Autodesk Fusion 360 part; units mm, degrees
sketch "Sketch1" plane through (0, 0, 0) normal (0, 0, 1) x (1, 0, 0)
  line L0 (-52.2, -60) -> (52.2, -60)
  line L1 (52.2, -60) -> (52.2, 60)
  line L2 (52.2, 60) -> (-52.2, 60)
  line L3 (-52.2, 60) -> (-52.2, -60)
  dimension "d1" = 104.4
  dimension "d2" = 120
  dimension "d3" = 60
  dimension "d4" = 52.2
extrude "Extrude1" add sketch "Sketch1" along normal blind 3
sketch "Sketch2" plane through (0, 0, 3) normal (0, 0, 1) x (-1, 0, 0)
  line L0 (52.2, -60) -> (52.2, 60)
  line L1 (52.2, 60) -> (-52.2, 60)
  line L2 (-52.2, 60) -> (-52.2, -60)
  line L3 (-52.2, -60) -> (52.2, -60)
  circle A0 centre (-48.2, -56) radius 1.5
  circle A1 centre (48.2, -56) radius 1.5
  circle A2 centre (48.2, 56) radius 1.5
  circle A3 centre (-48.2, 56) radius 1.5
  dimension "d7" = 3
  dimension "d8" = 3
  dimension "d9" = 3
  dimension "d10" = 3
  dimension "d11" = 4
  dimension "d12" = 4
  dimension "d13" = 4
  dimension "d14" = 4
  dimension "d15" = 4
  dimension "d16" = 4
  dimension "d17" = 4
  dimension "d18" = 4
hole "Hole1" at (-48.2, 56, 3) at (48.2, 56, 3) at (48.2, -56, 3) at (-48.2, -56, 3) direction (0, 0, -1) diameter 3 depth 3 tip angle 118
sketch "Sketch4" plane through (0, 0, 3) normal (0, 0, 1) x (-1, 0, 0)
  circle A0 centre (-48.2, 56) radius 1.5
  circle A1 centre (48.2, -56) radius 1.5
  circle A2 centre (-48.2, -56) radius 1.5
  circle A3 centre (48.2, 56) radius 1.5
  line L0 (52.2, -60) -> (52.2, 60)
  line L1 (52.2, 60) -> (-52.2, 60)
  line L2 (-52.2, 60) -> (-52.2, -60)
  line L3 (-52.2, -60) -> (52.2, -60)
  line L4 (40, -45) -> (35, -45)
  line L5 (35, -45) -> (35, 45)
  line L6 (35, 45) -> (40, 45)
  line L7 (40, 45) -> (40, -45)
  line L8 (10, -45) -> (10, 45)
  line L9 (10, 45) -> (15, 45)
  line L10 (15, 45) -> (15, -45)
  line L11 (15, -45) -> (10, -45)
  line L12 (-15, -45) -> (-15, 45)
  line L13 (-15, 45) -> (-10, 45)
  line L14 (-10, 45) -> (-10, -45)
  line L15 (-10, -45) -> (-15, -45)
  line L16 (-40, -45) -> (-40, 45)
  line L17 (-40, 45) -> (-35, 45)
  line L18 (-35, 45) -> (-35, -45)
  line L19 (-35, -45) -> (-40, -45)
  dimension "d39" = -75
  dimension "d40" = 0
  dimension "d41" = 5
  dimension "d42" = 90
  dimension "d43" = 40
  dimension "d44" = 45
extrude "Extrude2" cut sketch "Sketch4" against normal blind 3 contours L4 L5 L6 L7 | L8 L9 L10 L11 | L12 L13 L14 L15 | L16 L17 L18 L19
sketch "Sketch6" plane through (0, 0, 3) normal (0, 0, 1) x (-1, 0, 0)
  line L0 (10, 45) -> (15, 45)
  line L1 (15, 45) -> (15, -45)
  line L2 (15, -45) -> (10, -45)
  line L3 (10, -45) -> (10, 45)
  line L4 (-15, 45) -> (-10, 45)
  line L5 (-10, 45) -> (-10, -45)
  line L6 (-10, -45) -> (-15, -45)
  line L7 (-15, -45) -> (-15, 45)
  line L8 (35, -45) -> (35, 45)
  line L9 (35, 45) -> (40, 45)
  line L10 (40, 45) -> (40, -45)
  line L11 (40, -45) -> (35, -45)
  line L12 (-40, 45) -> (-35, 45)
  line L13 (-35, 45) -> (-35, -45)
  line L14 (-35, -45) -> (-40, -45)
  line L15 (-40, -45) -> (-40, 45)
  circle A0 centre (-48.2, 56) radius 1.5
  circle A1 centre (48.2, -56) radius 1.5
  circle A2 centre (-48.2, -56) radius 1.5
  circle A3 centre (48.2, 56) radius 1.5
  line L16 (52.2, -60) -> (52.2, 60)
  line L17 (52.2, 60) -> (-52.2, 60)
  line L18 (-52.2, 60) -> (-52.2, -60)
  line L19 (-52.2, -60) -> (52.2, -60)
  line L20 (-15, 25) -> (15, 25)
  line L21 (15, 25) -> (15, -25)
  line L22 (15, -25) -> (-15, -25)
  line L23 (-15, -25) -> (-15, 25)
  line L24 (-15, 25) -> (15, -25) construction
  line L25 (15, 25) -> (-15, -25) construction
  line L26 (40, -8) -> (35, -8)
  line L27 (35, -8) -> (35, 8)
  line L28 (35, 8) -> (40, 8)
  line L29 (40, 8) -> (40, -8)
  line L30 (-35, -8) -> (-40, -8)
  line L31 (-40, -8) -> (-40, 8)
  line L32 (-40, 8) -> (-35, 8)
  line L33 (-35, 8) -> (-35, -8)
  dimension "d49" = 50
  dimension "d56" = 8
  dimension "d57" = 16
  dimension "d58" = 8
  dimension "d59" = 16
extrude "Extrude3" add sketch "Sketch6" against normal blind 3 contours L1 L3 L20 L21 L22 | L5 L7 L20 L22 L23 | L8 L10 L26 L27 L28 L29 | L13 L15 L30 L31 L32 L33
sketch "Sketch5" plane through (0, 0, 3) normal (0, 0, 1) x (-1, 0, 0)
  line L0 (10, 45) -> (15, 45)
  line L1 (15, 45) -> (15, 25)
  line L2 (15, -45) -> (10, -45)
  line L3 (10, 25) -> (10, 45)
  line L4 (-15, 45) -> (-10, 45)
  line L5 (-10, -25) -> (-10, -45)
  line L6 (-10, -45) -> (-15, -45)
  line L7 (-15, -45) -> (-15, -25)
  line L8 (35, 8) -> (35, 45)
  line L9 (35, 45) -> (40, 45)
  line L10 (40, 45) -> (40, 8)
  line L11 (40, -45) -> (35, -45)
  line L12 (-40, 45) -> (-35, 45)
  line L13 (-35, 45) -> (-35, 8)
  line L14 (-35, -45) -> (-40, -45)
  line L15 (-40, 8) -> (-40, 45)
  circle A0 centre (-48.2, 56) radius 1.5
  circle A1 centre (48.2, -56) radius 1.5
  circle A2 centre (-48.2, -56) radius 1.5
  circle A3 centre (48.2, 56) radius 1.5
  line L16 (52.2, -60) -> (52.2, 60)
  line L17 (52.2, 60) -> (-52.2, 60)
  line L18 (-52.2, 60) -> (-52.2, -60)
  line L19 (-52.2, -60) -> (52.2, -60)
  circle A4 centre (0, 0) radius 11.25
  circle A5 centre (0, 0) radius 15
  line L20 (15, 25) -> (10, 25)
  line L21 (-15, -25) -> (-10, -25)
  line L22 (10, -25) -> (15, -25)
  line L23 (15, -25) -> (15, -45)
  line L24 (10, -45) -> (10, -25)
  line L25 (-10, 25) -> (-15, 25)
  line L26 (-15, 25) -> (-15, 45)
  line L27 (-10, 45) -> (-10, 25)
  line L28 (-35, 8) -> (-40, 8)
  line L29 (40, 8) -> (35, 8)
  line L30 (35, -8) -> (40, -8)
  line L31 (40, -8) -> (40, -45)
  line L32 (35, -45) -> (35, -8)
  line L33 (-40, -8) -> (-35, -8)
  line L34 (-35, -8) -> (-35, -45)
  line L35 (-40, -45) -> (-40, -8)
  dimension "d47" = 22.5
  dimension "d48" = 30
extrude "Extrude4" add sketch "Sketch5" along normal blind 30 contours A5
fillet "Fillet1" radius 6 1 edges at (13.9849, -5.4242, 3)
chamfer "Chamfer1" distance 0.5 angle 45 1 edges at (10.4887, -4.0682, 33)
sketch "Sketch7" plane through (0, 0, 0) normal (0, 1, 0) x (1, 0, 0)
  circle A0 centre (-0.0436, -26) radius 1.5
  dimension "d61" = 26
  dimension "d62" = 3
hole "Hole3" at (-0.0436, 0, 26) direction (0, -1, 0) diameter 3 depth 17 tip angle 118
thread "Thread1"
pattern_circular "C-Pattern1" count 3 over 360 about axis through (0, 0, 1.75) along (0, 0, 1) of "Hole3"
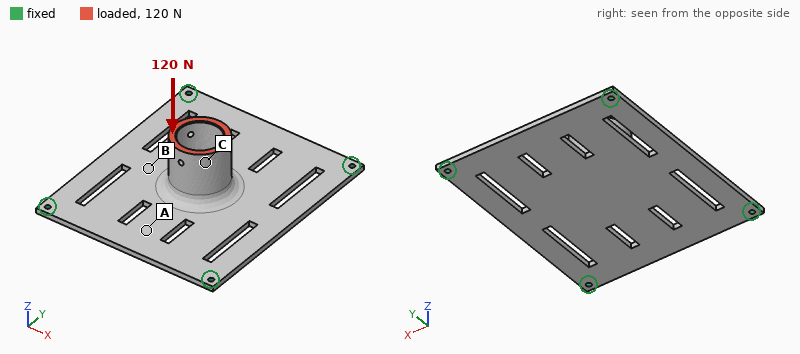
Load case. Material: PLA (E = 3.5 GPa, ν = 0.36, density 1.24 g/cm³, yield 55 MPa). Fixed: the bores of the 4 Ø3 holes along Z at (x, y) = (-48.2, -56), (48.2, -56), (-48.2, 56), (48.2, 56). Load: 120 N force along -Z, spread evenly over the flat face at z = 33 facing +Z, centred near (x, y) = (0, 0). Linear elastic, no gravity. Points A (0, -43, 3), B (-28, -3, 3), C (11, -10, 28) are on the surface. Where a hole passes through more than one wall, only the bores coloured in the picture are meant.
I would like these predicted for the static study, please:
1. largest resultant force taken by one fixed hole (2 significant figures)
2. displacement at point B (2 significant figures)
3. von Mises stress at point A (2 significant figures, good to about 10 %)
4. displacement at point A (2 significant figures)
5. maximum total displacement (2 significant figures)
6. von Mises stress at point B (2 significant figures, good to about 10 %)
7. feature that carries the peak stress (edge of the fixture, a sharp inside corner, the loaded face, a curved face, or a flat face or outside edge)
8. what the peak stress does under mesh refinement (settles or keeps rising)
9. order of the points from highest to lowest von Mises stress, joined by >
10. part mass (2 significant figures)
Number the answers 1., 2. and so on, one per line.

1. 31 N
2. 1.8 mm
3. 3.9 MPa
4. 1.2 mm
5. 1.9 mm
6. 7.2 MPa
7. edge of the fixture
8. keeps rising
9. B > A > C
10. 55 g
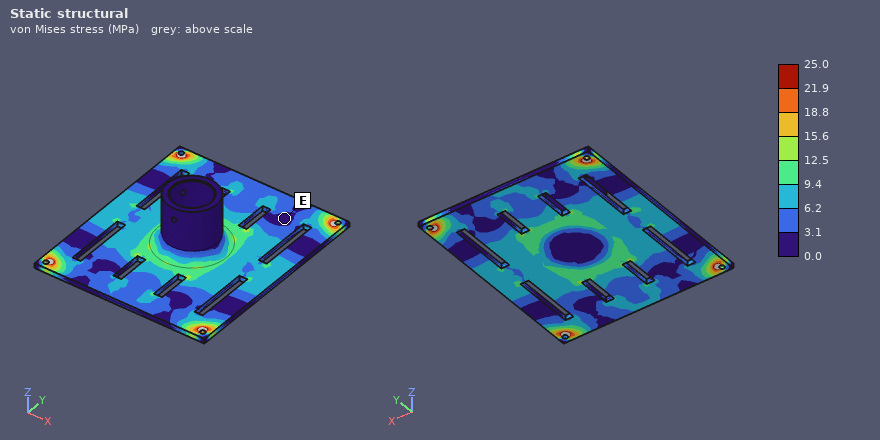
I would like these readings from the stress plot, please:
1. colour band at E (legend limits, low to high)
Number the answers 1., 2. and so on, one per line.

1. 0.0 to 3.1 MPa
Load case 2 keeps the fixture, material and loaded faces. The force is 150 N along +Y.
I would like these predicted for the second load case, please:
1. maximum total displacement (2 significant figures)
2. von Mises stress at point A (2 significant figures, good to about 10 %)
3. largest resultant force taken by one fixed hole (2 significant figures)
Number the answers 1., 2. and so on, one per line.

1. 1.6 mm
2. 5.0 MPa
3. 50 N
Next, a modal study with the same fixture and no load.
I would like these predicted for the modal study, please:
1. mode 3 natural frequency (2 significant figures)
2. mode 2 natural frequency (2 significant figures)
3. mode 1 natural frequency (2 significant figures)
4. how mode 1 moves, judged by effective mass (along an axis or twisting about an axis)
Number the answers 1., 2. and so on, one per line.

1. 440 Hz
2. 390 Hz
3. 220 Hz
4. along Z
